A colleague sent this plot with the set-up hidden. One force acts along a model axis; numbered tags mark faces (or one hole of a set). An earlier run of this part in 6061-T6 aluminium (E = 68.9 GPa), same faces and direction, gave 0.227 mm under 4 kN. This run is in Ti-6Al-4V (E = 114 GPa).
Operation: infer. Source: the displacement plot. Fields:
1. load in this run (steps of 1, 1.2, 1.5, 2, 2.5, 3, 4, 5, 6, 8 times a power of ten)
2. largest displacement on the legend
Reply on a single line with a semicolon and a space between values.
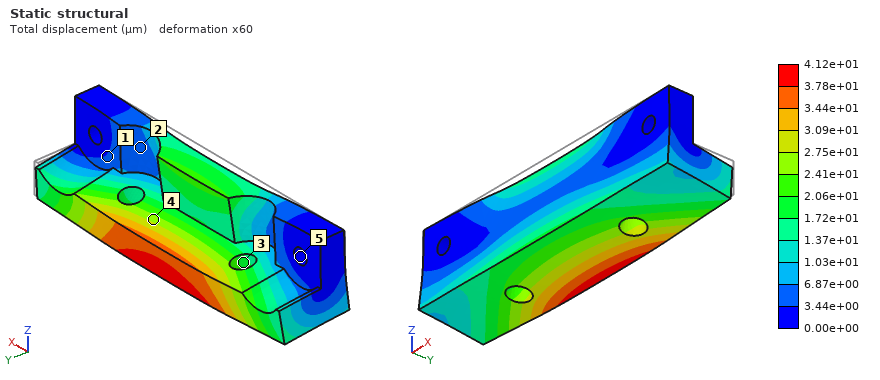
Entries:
1.2 kN; 4.12e+01 µm
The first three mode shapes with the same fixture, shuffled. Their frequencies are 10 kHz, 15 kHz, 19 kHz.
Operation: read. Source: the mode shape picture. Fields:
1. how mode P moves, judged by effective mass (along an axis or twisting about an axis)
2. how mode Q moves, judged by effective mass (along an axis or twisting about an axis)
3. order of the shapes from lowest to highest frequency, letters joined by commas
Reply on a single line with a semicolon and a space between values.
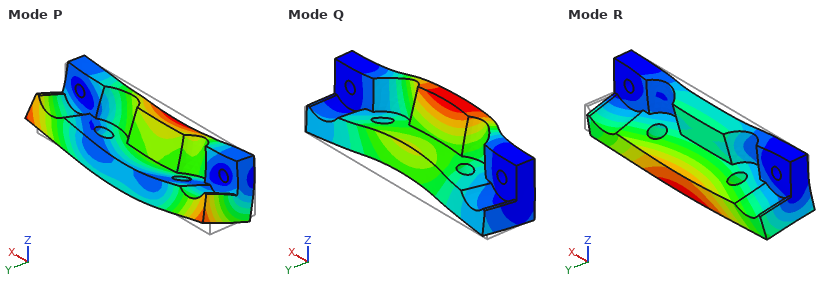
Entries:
along Z; along Y; R, Q, P
